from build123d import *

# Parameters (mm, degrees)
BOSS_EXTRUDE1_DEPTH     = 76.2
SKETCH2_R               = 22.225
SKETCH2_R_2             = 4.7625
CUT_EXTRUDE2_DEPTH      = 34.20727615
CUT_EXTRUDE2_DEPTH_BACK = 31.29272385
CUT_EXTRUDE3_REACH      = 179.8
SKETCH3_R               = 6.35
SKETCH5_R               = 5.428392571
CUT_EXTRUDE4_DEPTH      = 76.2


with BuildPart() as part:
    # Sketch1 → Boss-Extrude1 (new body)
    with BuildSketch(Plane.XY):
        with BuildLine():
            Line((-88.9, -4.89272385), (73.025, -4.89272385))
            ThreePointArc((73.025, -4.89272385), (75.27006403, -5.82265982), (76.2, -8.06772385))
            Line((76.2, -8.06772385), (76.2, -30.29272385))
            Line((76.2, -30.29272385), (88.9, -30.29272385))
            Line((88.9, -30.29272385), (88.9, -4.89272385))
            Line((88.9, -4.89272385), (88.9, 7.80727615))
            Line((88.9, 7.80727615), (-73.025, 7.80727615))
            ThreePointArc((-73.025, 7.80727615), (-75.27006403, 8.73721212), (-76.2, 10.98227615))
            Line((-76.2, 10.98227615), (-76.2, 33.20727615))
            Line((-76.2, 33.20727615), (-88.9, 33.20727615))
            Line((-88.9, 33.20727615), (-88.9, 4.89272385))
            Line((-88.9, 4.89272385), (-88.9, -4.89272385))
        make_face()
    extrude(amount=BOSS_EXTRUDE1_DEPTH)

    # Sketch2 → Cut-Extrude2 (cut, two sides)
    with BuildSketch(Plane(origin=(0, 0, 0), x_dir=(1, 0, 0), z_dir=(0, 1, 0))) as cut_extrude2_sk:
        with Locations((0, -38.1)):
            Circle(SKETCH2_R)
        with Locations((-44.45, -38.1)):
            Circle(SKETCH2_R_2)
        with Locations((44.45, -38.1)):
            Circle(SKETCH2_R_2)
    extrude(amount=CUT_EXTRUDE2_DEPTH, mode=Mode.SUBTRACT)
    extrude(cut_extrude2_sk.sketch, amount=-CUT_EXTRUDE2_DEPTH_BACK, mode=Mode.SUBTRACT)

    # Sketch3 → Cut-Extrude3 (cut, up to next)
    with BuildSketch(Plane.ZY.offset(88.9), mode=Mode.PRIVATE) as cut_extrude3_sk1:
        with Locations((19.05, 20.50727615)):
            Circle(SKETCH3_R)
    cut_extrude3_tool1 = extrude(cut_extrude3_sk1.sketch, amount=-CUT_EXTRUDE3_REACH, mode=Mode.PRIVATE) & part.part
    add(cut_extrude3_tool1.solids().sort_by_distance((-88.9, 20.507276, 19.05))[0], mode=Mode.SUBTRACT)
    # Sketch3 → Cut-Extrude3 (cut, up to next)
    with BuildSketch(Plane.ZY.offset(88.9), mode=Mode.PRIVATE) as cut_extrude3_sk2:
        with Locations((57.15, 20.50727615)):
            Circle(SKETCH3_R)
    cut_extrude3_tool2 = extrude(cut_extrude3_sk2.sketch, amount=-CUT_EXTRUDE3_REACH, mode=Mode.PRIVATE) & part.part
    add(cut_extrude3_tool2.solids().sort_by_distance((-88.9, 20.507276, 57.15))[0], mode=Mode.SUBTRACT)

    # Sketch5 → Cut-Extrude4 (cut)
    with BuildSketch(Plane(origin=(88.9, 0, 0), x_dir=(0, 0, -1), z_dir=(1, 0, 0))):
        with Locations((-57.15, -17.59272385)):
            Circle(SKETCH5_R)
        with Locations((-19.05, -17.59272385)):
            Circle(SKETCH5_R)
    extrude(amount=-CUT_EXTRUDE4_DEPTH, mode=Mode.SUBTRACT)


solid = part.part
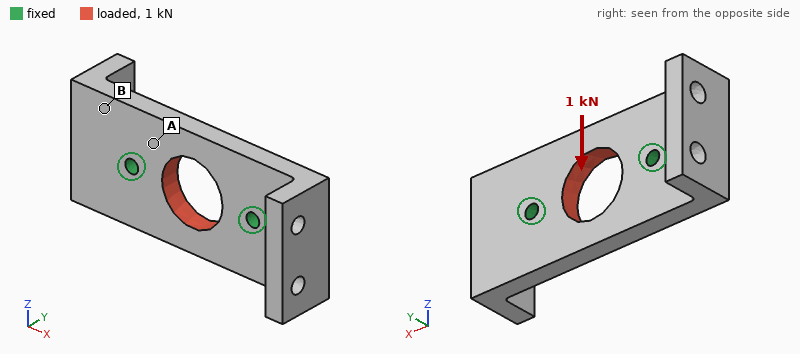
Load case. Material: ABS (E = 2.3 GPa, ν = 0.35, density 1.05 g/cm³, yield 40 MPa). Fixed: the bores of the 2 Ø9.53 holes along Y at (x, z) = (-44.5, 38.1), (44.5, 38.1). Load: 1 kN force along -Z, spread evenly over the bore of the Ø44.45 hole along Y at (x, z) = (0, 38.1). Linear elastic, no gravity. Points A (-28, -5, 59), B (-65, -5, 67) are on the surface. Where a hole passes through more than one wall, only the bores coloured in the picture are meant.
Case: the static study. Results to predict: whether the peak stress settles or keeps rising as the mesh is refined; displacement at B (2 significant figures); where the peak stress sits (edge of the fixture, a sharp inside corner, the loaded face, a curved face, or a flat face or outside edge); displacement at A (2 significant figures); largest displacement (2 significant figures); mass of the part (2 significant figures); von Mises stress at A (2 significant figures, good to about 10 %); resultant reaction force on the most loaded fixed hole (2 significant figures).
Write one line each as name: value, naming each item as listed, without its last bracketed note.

whether the peak stress settles or keeps rising as the mesh is refined: keeps rising
displacement at B: 11 µm
where the peak stress sits: edge of the fixture
displacement at A: 19 µm
largest displacement: 42 µm
mass of the part: 200 g
von Mises stress at A: 0.98 MPa
resultant reaction force on the most loaded fixed hole: 500 N
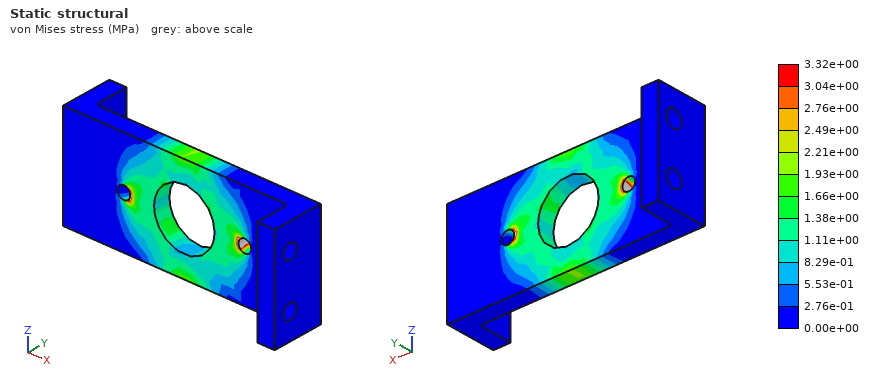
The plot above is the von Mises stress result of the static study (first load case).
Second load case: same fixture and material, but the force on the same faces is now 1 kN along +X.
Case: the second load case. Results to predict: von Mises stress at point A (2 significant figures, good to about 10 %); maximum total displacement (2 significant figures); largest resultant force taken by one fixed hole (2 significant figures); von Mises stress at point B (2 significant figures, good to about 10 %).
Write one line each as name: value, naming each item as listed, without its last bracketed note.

von Mises stress at point A: 0.64 MPa
maximum total displacement: 20 µm
largest resultant force taken by one fixed hole: 500 N
von Mises stress at point B: 0.18 MPa
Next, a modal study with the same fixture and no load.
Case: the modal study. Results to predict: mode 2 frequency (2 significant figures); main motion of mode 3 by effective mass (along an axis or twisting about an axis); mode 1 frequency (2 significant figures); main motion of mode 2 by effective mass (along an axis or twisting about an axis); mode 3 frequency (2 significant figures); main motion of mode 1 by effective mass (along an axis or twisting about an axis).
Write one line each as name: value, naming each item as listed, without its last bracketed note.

mode 2 frequency: 750 Hz
main motion of mode 3 by effective mass: twisting about X
mode 1 frequency: 720 Hz
main motion of mode 2 by effective mass: twisting about Z
mode 3 frequency: 860 Hz
main motion of mode 1 by effective mass: along Y
